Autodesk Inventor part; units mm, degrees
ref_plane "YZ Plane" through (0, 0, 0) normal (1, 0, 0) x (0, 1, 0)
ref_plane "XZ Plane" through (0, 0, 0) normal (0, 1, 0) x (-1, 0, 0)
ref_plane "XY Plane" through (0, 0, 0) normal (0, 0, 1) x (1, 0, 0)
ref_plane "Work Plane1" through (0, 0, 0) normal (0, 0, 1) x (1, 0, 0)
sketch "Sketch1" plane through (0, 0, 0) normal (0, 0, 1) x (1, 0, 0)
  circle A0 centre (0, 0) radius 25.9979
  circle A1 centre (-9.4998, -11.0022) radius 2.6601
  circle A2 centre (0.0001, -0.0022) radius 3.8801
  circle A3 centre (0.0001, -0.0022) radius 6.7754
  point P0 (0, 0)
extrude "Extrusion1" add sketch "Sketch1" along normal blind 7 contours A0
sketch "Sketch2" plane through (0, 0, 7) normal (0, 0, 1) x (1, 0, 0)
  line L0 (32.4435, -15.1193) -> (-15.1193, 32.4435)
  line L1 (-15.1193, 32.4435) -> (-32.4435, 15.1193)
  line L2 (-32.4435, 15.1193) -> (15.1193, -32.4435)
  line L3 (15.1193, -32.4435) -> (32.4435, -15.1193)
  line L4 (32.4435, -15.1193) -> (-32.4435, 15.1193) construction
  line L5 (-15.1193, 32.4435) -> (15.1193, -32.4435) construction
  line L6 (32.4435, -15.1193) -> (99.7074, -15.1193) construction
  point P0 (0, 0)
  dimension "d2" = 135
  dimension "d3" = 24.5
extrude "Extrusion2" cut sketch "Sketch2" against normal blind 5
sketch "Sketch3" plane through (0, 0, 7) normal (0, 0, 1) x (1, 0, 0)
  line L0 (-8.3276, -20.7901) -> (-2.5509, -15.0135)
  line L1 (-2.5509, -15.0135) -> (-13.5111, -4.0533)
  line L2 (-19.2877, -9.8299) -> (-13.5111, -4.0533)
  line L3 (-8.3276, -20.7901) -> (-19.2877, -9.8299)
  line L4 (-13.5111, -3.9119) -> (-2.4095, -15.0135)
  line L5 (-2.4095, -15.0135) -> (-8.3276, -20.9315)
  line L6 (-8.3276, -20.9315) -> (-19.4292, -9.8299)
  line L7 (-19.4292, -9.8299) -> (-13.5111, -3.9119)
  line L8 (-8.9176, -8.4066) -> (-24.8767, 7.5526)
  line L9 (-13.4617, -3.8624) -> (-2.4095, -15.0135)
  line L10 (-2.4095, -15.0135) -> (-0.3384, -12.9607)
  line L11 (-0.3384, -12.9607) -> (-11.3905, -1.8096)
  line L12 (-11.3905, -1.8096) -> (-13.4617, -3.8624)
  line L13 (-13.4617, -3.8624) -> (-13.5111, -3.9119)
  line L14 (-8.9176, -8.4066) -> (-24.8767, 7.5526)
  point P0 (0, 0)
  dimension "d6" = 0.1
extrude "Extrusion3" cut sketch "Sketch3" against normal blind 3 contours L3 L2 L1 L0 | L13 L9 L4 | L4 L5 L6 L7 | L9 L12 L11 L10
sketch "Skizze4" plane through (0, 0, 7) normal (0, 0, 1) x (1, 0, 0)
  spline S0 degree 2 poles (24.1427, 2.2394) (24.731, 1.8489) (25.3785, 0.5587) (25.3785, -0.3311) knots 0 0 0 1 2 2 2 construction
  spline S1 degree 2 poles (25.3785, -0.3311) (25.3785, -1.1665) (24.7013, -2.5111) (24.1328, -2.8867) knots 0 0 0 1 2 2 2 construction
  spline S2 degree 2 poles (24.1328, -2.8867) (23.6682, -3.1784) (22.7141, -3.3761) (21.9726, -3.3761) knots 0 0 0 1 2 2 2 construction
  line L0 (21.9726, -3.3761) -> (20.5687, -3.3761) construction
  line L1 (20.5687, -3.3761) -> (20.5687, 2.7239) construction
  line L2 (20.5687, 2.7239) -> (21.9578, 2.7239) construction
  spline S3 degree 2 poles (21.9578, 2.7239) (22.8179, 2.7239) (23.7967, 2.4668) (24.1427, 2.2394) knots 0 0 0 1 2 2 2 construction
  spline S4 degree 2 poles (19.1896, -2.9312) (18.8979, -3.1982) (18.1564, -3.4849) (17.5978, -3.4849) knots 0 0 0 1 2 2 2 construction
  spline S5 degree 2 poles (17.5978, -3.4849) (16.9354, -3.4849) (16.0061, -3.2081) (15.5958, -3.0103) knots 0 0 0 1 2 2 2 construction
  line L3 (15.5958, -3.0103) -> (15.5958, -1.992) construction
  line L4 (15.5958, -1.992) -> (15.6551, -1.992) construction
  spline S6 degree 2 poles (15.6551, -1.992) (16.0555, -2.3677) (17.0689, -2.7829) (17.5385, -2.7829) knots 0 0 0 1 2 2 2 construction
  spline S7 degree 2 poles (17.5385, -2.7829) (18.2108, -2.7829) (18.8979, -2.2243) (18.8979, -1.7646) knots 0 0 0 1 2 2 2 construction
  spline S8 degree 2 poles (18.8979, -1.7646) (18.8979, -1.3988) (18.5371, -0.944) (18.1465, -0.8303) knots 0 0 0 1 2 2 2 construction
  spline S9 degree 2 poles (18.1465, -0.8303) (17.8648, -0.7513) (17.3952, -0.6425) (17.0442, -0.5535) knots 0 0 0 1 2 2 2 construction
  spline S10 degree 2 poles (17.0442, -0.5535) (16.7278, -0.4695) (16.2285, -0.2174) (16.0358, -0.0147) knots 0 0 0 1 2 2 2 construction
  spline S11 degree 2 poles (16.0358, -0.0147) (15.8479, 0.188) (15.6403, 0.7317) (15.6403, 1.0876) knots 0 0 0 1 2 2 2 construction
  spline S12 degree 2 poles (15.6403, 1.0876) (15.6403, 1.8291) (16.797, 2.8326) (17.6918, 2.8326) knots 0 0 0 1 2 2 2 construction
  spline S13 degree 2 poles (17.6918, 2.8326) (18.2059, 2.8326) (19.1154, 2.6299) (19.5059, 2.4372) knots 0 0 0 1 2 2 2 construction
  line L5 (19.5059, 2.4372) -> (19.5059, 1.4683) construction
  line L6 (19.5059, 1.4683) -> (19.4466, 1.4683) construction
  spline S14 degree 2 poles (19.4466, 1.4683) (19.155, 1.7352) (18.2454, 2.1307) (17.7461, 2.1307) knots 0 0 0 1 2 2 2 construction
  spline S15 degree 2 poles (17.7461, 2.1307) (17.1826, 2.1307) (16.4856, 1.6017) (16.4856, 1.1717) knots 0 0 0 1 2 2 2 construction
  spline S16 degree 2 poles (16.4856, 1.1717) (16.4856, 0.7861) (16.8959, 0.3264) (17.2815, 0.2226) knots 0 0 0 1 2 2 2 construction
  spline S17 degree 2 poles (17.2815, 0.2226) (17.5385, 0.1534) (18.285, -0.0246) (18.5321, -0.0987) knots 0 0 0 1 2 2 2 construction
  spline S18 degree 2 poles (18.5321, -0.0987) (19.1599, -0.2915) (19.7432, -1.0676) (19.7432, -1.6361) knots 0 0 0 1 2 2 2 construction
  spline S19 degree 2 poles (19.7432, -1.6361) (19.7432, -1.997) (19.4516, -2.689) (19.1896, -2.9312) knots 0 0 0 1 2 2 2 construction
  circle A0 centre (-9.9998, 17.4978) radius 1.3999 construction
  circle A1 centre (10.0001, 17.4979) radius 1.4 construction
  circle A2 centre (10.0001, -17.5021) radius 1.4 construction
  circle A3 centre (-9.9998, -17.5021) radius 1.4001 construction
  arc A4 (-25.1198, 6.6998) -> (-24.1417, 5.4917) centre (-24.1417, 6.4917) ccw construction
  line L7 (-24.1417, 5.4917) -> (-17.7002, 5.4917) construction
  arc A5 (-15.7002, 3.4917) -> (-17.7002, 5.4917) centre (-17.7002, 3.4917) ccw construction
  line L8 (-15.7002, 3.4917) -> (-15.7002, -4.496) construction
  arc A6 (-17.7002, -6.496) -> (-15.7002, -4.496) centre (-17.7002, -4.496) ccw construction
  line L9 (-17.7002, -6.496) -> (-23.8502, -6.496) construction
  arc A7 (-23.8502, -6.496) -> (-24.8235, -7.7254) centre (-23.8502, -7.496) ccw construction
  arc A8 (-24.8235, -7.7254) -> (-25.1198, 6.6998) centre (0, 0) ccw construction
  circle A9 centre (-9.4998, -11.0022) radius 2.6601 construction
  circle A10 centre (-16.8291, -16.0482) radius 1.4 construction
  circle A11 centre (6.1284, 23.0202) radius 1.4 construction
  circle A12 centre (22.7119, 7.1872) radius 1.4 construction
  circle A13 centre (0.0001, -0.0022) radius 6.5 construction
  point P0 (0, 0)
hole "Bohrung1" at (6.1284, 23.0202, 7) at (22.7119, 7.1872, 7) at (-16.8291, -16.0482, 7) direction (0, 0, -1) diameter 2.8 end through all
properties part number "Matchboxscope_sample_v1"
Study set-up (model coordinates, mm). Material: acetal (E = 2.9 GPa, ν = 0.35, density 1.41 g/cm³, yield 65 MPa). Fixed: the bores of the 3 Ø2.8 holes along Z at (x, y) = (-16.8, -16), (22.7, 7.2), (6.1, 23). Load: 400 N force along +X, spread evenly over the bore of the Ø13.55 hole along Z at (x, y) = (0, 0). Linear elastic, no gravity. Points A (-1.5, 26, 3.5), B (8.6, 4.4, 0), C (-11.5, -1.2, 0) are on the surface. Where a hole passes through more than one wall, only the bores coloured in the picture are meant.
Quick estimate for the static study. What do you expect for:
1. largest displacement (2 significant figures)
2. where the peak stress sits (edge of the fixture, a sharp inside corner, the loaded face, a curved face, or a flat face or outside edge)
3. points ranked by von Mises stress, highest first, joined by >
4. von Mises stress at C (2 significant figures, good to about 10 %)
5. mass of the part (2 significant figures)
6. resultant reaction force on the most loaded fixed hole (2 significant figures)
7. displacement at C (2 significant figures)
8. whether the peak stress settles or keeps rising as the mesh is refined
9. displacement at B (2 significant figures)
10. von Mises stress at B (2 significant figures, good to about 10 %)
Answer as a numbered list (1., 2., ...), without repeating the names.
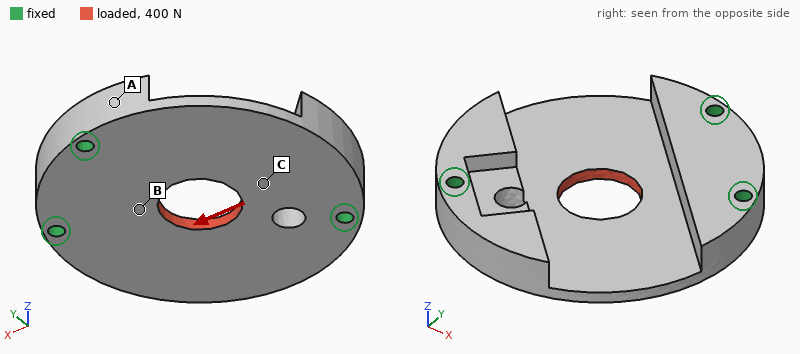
1. 67 µm
2. edge of the fixture
3. B > C > A
4. 3.3 MPa
5. 11 g
6. 170 N
7. 42 µm
8. keeps rising
9. 30 µm
10. 6.2 MPa
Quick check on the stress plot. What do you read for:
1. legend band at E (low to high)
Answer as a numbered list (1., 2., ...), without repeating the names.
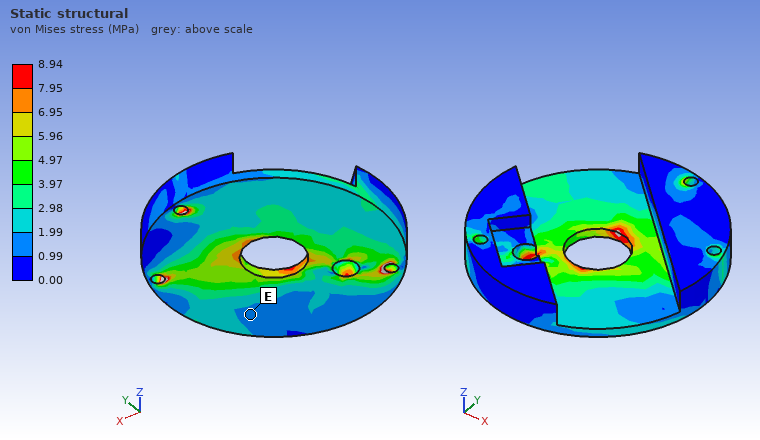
1. 0.99 to 1.99 MPa
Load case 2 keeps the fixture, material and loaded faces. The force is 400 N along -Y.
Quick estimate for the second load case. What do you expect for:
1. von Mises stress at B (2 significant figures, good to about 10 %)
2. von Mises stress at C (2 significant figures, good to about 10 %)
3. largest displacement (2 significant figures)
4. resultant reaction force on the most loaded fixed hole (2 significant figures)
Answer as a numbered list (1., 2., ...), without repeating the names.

1. 5.5 MPa
2. 2.5 MPa
3. 74 µm
4. 160 N
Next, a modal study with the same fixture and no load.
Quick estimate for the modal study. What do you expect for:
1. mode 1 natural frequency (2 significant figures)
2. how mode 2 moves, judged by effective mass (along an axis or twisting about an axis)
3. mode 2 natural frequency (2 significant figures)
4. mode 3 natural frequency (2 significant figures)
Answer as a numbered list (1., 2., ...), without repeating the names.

1. 2000 Hz
2. along Z
3. 2300 Hz
4. 4000 Hz
